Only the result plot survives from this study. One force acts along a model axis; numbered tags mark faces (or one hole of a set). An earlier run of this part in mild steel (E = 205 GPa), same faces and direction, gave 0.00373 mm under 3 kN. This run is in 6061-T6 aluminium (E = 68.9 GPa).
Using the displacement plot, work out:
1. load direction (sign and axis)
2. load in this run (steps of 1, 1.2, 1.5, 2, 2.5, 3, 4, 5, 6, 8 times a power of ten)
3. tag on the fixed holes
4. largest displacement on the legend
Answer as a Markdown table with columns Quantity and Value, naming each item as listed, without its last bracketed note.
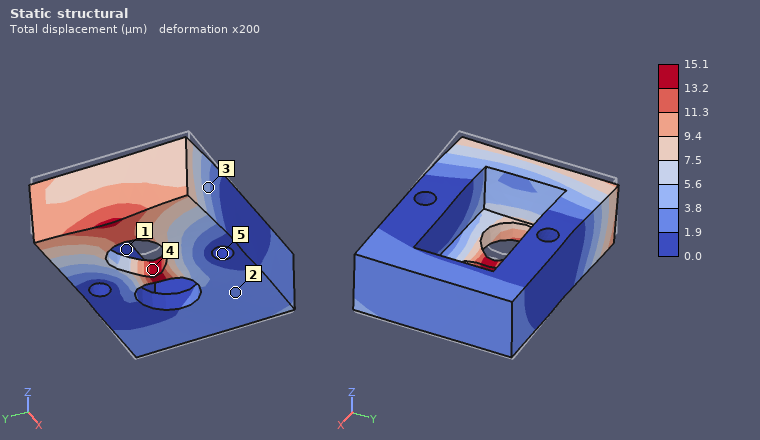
| Quantity | Value |
|---|---|
| load direction | +X |
| load in this run | 4 kN |
| tag on the fixed holes | 5 |
| largest displacement on the legend | 15.1 µm |
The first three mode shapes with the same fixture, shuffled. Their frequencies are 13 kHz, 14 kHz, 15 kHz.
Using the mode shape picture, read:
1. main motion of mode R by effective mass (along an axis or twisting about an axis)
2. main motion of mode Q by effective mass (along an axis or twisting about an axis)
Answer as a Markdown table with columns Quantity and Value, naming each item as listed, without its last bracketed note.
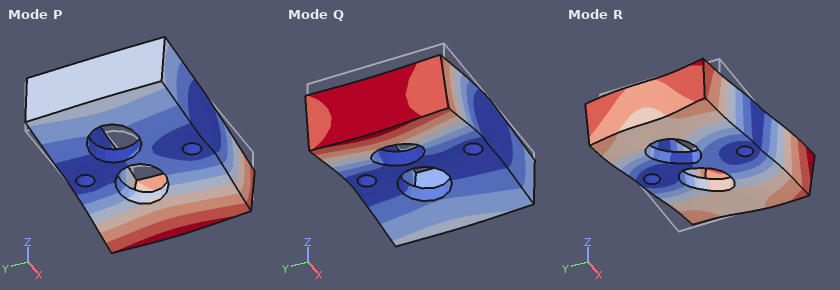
| Quantity | Value |
|---|---|
| main motion of mode R by effective mass | twisting about Z |
| main motion of mode Q by effective mass | along Z |
